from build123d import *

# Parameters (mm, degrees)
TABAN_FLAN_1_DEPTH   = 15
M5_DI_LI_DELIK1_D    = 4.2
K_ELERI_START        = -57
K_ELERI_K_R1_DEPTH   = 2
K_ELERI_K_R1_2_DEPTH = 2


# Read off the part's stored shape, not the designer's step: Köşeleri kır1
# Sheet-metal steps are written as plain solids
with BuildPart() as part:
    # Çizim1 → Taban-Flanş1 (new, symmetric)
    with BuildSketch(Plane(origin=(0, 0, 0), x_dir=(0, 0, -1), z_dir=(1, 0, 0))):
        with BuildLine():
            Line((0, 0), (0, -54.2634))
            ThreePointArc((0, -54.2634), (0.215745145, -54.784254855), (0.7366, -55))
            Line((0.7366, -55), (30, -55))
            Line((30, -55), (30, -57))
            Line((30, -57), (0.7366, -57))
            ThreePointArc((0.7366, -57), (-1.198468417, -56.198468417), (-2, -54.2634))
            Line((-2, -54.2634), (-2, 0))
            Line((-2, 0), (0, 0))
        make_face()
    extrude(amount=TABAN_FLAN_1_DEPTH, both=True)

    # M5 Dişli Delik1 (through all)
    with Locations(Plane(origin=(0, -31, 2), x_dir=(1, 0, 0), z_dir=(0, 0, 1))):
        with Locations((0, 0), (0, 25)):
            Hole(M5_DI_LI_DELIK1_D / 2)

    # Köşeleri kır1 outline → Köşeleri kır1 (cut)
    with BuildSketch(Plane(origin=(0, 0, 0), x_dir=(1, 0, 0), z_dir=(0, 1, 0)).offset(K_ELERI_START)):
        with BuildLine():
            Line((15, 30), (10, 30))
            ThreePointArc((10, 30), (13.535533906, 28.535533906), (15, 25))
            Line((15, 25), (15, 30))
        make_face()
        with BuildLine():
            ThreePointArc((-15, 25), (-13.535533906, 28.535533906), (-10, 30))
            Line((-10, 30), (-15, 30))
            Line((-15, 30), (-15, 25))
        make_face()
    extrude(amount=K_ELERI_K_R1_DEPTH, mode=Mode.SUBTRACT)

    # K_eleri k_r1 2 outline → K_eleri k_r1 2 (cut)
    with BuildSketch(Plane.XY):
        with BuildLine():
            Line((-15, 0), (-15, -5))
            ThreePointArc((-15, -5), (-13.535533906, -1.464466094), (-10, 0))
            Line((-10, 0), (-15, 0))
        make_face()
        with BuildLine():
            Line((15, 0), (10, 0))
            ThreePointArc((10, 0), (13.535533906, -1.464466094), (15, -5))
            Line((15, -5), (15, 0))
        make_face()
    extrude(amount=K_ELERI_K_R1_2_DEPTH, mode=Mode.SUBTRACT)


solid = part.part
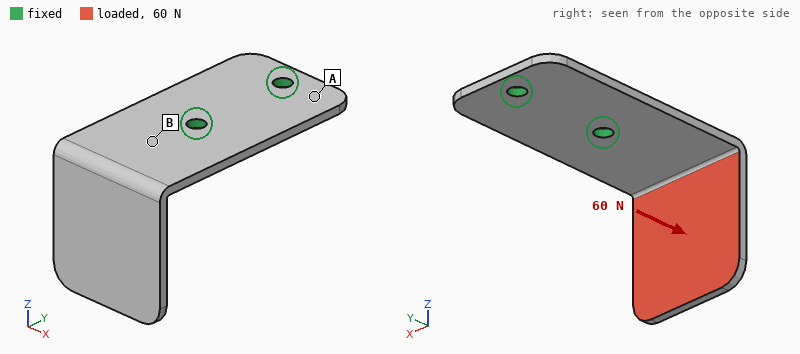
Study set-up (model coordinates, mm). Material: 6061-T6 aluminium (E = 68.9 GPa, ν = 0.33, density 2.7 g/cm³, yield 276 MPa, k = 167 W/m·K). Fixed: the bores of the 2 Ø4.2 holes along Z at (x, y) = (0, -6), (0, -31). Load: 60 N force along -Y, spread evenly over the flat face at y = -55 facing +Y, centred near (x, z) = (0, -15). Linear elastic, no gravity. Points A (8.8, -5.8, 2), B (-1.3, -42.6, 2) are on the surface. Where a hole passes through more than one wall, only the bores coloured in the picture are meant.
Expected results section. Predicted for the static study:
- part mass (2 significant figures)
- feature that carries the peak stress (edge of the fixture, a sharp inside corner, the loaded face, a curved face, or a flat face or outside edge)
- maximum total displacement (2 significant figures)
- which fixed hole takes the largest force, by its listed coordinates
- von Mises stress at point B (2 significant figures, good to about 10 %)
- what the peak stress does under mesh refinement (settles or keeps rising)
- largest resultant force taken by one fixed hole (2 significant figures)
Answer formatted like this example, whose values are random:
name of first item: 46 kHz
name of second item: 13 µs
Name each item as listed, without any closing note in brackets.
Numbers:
part mass: 14 g
feature that carries the peak stress: edge of the fixture
maximum total displacement: 0.70 mm
which fixed hole takes the largest force, by its listed coordinates: (0, -31)
von Mises stress at point B: 41 MPa
what the peak stress does under mesh refinement: keeps rising
largest resultant force taken by one fixed hole: 49 N
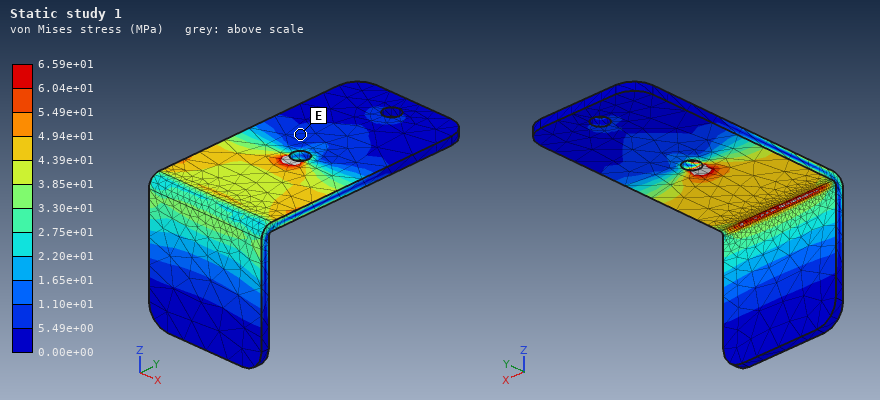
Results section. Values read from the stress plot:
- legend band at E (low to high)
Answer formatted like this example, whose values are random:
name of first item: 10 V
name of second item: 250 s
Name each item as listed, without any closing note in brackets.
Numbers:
legend band at E: 5.49e+00 to 1.10e+01 MPa
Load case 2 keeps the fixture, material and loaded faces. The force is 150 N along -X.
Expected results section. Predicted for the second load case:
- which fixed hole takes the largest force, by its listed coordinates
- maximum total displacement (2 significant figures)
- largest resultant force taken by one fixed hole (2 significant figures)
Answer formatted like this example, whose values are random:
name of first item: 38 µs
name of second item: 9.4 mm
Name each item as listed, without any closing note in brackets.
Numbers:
which fixed hole takes the largest force, by its listed coordinates: (0, -31)
maximum total displacement: 0.86 mm
largest resultant force taken by one fixed hole: 270 N
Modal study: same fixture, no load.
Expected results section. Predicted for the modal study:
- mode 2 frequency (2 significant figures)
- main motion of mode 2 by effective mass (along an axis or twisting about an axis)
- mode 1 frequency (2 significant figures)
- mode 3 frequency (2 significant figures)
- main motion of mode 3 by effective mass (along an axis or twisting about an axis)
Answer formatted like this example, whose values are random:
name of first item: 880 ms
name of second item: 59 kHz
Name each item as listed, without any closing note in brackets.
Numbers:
mode 2 frequency: 1100 Hz
main motion of mode 2 by effective mass: along X
mode 1 frequency: 720 Hz
mode 3 frequency: 2000 Hz
main motion of mode 3 by effective mass: along Z
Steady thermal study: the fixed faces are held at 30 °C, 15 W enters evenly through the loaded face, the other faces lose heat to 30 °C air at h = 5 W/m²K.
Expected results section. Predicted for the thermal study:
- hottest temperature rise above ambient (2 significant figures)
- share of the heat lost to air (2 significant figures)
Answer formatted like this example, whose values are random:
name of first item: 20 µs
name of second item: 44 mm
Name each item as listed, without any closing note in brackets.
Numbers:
hottest temperature rise above ambient: 63 K
share of the heat lost to air: 3.4 %
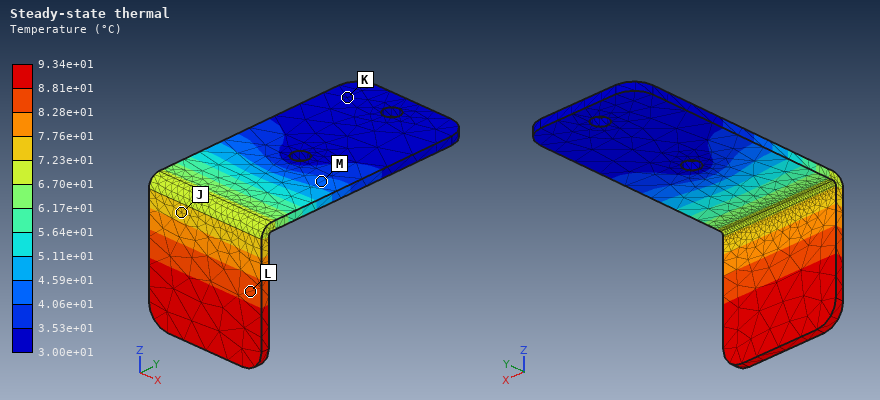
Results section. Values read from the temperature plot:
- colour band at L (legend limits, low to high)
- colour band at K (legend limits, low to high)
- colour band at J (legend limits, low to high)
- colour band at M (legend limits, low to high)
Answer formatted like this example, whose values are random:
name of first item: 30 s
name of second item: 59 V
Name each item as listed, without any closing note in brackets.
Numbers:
colour band at L: 8.28e+01 to 8.81e+01 °C
colour band at K: 3.00e+01 to 3.53e+01 °C
colour band at J: 7.23e+01 to 7.76e+01 °C
colour band at M: 4.06e+01 to 4.59e+01 °C
